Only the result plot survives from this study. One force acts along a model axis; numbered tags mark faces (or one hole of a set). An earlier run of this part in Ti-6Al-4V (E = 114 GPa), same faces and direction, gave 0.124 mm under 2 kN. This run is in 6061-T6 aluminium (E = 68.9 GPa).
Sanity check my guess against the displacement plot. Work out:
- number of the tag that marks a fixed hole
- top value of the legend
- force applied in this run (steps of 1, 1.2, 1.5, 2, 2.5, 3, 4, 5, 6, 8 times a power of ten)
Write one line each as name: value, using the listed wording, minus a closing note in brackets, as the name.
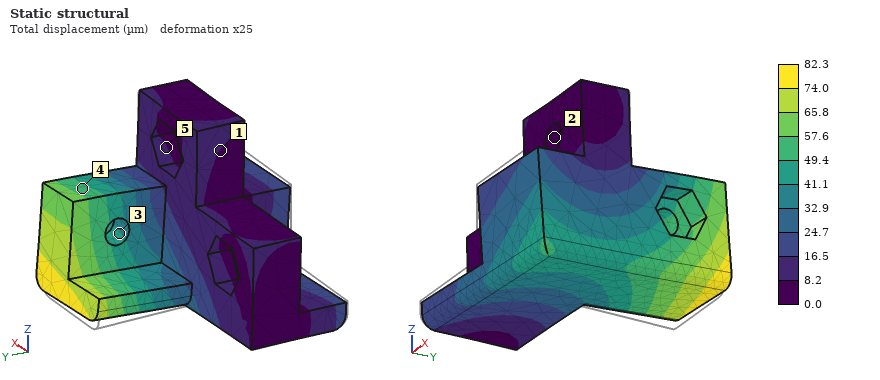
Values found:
number of the tag that marks a fixed hole: 2
top value of the legend: 82.3 µm
force applied in this run: 800 N
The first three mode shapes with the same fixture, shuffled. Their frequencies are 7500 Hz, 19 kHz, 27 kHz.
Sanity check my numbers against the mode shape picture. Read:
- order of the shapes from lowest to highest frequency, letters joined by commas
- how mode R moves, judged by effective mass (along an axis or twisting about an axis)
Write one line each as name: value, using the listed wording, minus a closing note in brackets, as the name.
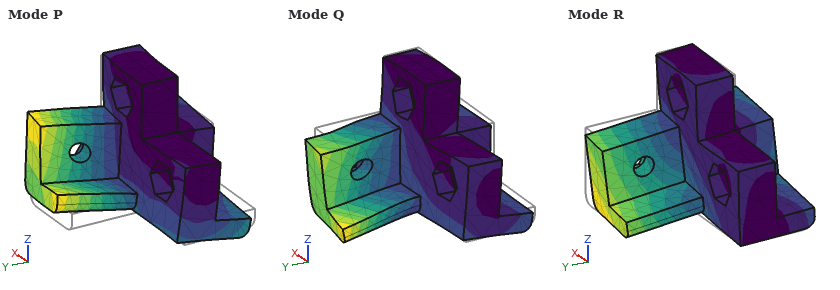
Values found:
order of the shapes from lowest to highest frequency, letters joined by commas: R, P, Q
how mode R moves, judged by effective mass: along Y
